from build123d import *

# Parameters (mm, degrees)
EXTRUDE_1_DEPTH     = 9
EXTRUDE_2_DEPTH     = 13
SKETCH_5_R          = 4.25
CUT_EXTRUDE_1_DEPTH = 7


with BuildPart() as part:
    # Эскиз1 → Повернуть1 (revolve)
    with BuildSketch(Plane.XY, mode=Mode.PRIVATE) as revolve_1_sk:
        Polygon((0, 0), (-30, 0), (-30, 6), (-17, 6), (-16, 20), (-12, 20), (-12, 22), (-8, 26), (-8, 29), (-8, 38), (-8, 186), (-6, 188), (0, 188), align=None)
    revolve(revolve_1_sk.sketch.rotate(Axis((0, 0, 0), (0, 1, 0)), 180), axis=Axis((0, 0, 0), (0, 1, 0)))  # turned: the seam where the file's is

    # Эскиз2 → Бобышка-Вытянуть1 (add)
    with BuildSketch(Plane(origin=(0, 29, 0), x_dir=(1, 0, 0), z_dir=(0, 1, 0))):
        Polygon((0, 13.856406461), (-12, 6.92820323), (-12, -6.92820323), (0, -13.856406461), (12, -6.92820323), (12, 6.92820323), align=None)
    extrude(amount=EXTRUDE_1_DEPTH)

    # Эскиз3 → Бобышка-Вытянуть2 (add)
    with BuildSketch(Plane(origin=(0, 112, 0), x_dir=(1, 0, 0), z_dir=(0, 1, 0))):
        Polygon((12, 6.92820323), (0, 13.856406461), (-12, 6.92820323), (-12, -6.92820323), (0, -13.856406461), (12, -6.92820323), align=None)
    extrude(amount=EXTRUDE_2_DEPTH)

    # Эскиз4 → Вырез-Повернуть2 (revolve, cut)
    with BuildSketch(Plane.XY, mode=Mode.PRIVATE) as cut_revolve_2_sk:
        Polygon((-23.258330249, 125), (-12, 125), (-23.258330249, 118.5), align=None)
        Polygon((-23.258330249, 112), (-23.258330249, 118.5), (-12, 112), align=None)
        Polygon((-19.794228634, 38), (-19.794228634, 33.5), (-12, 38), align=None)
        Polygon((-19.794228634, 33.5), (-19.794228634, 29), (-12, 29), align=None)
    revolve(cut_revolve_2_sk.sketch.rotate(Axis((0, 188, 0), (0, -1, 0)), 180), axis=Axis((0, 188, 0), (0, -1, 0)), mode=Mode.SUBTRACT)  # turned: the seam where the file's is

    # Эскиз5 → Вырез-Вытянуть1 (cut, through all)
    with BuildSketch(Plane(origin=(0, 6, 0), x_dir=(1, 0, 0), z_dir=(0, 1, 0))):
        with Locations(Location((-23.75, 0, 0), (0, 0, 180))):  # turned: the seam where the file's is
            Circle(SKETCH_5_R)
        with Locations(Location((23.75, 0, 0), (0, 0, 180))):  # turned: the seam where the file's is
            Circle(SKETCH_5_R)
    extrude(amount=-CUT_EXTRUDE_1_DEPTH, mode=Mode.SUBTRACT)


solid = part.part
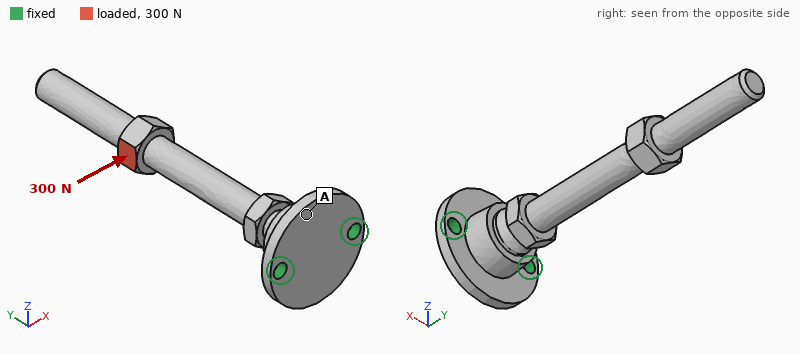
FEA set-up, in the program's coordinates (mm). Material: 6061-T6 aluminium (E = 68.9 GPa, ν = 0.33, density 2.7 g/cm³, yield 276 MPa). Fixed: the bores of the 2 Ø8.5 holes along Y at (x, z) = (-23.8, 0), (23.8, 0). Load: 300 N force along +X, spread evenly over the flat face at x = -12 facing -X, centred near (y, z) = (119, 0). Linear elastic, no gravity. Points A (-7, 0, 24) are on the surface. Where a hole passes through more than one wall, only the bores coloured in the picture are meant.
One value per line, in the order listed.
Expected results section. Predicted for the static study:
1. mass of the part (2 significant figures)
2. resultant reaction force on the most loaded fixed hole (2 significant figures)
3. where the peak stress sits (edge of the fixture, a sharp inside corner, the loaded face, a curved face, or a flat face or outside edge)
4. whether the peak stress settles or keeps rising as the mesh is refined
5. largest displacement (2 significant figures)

190 g
930 N
a sharp inside corner
keeps rising
0.82 mm
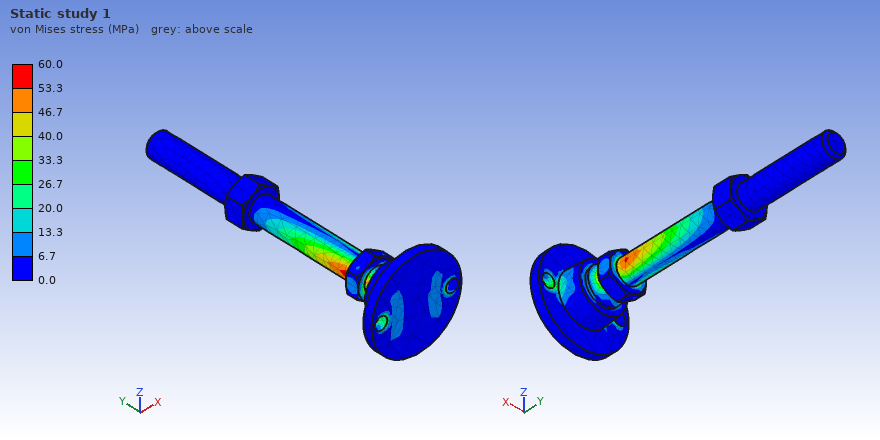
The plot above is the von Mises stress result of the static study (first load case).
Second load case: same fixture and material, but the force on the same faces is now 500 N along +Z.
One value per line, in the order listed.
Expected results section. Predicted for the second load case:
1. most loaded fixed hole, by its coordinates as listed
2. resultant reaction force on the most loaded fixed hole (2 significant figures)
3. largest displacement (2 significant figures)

(-23.8, 0)
370 N
1.9 mm
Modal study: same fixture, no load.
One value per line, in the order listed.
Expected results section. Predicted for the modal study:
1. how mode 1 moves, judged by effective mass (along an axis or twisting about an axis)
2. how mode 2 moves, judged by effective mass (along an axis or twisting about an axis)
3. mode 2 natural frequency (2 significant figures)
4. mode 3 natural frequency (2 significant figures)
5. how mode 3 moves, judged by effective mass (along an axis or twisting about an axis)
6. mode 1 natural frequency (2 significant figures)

along Z
along X
400 Hz
1900 Hz
along Z
340 Hz
